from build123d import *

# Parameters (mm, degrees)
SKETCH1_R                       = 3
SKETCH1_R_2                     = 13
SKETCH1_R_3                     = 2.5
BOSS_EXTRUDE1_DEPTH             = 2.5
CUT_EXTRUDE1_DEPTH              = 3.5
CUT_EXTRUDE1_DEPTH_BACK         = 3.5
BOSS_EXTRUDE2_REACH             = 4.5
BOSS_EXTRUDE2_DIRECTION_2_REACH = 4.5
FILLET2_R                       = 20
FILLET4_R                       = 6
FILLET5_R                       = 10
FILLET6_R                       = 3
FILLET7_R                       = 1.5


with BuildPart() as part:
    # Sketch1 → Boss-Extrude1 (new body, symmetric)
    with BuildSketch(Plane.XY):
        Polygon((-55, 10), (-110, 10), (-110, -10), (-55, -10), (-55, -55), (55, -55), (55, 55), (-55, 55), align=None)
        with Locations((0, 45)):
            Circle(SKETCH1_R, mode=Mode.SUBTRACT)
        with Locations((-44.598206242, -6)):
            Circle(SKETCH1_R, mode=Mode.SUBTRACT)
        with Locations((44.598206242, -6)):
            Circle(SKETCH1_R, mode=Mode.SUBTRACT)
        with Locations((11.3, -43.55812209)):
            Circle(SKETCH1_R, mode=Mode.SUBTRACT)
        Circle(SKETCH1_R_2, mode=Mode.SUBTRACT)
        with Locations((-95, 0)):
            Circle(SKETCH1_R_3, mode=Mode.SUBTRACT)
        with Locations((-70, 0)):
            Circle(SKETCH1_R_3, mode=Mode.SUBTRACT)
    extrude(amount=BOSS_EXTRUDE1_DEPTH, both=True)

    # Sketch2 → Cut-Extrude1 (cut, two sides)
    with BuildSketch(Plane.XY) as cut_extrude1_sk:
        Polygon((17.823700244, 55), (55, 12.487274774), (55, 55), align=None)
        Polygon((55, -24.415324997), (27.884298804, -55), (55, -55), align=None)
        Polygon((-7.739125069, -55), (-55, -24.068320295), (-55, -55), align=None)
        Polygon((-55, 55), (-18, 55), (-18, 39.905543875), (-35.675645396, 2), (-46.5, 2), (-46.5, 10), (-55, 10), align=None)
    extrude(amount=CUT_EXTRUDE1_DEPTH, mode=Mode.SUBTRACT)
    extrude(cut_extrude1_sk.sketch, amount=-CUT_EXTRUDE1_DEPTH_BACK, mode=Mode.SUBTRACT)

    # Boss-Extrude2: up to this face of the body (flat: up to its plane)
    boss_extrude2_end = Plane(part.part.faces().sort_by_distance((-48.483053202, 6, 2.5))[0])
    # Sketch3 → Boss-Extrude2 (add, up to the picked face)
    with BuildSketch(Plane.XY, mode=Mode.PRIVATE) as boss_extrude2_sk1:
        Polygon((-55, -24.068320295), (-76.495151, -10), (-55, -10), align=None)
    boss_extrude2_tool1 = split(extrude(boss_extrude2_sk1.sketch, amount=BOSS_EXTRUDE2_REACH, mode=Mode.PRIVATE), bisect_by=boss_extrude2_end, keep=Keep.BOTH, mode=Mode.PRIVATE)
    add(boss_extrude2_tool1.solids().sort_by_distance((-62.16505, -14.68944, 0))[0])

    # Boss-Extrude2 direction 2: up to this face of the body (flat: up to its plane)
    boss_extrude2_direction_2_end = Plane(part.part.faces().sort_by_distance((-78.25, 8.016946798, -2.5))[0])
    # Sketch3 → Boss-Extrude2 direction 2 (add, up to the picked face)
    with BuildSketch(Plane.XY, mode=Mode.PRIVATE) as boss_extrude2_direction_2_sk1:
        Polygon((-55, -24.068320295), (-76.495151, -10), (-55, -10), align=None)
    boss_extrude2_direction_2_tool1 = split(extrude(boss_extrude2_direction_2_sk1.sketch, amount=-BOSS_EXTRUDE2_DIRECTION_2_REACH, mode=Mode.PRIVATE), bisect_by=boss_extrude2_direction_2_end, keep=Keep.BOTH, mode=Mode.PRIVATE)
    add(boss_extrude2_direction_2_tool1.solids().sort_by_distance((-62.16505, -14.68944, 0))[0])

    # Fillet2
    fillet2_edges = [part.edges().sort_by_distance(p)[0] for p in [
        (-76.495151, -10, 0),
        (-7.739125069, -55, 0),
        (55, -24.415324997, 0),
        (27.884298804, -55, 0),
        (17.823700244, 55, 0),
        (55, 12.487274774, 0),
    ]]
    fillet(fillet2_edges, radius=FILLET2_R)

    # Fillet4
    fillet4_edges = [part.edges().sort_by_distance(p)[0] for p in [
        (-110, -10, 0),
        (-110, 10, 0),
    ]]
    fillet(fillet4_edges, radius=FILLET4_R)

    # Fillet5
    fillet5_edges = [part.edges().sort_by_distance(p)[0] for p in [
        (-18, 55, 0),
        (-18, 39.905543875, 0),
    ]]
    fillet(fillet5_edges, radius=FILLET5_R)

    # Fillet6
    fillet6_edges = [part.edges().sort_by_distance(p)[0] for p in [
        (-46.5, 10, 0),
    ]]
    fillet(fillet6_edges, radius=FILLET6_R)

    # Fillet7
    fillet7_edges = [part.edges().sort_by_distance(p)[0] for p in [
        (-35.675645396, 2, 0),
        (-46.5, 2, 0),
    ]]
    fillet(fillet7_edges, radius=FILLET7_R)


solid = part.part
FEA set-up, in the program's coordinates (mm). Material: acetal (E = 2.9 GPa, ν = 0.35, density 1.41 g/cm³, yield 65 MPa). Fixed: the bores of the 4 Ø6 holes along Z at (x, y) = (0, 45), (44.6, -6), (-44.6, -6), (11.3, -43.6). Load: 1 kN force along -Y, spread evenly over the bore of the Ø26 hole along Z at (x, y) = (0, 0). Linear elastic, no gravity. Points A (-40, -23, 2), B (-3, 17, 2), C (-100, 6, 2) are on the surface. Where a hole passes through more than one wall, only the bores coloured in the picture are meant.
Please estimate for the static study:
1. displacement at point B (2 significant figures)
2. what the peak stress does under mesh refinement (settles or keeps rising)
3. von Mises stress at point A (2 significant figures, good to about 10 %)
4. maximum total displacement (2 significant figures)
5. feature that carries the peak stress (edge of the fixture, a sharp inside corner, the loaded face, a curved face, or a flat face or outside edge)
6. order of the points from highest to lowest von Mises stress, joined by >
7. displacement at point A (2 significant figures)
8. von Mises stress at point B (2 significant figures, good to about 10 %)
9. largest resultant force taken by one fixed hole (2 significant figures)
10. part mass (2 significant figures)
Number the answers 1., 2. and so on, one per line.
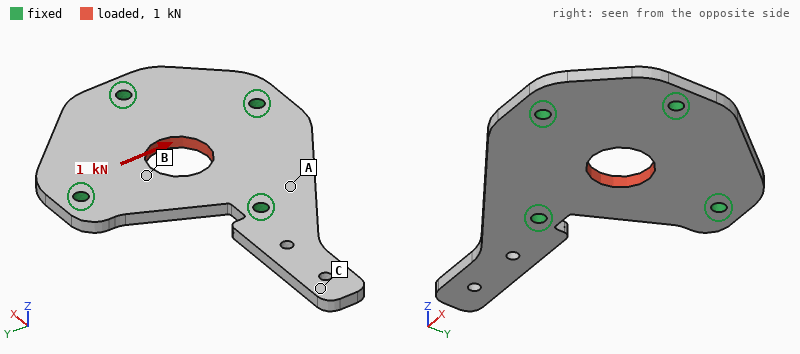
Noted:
1. 31 µm
2. keeps rising
3. 1.4 MPa
4. 48 µm
5. edge of the fixture
6. B > A > C
7. 16 µm
8. 3.2 MPa
9. 360 N
10. 64 g
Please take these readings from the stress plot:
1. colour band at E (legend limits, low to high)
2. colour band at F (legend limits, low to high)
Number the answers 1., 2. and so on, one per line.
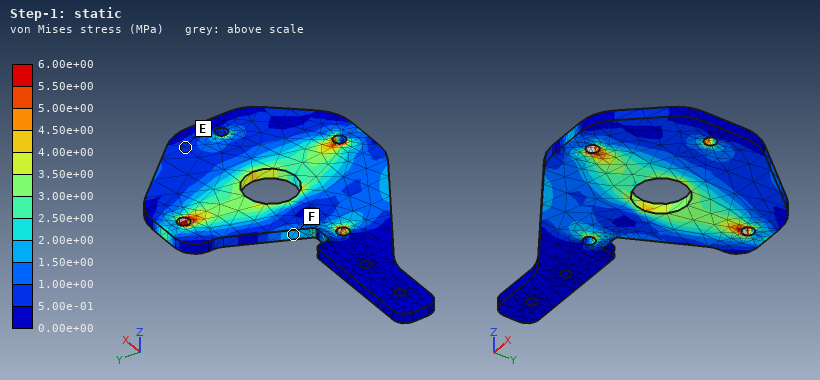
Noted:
1. 5.00e-01 to 1.00e+00 MPa
2. 1.50e+00 to 2.00e+00 MPa
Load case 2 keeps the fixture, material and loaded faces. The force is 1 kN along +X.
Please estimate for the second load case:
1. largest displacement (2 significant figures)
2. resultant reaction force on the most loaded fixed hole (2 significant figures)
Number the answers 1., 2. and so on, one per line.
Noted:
1. 52 µm
2. 340 N
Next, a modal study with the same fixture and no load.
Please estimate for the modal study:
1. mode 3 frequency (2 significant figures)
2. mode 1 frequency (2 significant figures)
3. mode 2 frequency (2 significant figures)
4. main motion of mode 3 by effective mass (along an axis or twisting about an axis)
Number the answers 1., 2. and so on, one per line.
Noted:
1. 1300 Hz
2. 320 Hz
3. 1300 Hz
4. along Z
